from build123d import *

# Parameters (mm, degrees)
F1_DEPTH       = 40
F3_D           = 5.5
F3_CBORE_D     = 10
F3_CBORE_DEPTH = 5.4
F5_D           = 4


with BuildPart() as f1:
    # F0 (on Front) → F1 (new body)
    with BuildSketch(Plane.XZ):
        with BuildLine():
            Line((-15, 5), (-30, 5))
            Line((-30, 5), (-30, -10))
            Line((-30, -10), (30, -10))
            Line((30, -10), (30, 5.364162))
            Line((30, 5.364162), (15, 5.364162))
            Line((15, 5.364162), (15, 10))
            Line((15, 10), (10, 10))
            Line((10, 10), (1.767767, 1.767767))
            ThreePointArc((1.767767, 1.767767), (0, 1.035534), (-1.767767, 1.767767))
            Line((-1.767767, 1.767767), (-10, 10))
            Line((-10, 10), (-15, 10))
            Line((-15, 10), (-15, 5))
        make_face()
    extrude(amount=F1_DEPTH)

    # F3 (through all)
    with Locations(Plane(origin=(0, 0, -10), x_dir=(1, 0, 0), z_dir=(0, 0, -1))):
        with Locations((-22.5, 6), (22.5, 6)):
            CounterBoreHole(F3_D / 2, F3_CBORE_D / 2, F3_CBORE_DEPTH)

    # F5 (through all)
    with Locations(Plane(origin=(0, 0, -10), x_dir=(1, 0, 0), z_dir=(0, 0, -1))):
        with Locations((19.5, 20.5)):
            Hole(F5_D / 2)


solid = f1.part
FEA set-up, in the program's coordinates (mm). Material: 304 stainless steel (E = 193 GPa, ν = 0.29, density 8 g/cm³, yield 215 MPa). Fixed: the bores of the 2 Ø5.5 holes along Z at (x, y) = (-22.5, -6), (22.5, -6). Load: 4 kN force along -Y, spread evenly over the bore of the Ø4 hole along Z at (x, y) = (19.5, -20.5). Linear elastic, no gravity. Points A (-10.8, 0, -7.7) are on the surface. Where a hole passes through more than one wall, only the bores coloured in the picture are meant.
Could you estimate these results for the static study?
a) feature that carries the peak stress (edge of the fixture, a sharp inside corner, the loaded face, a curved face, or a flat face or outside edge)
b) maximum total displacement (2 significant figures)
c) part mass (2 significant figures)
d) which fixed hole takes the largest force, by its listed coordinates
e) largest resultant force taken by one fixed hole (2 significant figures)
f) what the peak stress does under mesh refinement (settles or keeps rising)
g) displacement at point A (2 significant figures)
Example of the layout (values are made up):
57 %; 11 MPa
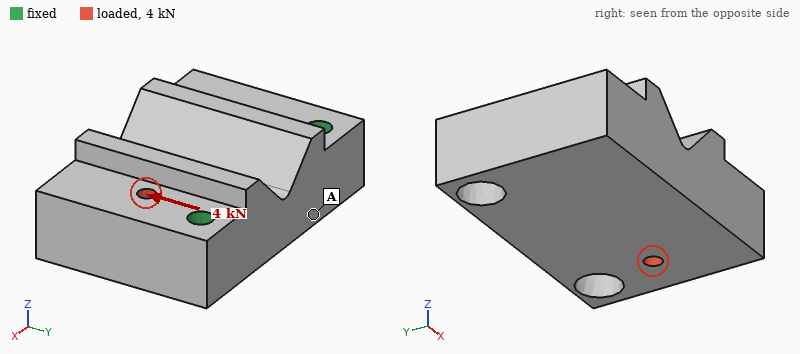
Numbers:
edge of the fixture; 4.4 µm; 290 g; (22.5, -6); 3.7 kN; keeps rising; 1.0 µm
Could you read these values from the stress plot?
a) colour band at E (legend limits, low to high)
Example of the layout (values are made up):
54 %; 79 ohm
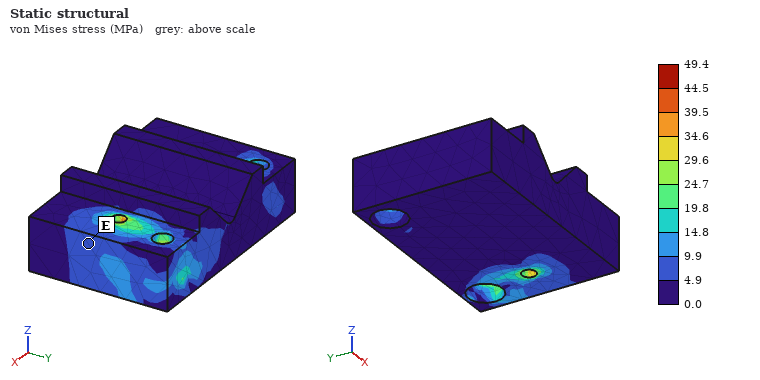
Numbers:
4.9 to 9.9 MPa
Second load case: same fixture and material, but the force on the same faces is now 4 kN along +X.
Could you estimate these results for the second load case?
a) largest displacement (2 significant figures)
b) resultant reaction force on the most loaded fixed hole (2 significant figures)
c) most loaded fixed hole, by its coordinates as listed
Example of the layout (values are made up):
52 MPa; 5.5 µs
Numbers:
2.6 µm; 2.7 kN; (22.5, -6)
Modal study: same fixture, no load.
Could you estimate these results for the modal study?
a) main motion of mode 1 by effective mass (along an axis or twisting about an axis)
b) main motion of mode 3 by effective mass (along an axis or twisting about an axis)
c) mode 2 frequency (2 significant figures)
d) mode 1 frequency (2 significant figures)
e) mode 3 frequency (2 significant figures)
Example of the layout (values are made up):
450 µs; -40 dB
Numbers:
along Z; along X; 11 kHz; 5000 Hz; 15 kHz
